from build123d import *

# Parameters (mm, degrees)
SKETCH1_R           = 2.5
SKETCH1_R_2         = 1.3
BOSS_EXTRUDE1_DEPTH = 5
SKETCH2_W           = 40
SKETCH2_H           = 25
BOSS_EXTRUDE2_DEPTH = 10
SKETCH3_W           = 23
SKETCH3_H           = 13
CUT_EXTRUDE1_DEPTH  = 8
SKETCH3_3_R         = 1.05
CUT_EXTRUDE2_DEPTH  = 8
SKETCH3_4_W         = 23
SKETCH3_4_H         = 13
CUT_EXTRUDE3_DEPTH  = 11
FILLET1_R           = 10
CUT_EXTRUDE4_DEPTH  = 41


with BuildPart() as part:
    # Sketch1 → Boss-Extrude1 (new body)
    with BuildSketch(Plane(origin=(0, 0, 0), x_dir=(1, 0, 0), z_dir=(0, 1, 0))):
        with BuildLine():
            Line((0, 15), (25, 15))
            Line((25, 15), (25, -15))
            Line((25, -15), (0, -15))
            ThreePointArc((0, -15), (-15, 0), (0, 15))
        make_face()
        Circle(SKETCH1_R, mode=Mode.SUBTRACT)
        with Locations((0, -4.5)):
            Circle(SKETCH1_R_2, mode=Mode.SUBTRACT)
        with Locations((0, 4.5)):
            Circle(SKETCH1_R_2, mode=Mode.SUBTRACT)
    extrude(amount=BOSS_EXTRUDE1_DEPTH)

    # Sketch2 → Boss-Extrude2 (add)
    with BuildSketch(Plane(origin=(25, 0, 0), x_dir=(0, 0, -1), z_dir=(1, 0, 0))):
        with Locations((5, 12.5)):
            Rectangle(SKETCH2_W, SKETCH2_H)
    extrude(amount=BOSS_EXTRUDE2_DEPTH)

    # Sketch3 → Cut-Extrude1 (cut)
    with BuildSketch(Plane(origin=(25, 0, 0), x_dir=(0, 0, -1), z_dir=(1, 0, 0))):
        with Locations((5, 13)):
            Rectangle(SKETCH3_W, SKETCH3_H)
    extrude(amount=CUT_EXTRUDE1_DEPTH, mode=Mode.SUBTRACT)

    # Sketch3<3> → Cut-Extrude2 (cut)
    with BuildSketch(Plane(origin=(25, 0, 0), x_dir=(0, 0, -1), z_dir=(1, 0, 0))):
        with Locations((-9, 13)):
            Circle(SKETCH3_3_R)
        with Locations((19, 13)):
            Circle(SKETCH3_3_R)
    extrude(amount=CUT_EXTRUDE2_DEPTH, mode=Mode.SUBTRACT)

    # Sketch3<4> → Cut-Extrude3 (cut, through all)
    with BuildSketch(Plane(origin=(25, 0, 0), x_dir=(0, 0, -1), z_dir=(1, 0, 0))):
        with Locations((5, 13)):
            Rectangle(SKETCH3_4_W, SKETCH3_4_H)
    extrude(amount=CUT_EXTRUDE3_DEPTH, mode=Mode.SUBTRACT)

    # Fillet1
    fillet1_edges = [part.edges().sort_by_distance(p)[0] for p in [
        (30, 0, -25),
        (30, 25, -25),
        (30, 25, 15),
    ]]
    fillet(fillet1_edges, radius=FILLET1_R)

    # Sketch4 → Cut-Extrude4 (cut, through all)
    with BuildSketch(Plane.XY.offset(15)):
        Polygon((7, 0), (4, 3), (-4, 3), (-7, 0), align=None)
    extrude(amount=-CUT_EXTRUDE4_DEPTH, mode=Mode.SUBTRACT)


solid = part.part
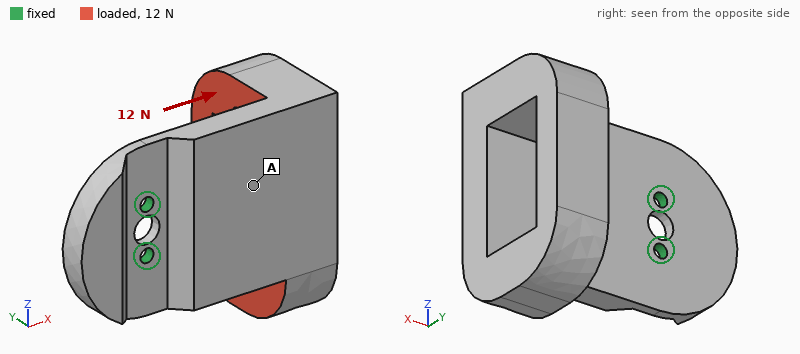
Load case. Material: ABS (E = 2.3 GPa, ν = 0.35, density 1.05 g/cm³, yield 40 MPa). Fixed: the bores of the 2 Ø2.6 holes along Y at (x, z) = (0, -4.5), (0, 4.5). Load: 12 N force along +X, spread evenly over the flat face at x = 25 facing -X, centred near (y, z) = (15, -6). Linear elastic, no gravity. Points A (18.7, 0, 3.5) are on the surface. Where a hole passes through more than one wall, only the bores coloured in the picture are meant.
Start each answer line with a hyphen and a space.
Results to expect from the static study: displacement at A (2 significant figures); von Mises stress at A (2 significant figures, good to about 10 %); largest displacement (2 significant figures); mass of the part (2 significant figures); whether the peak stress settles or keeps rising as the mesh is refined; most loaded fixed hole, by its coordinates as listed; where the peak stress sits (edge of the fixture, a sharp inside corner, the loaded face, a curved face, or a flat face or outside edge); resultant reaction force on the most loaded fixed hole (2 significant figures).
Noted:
- 0.28 mm
- 0.98 MPa
- 0.74 mm
- 11 g
- keeps rising
- (0, -4.5)
- edge of the fixture
- 13 N
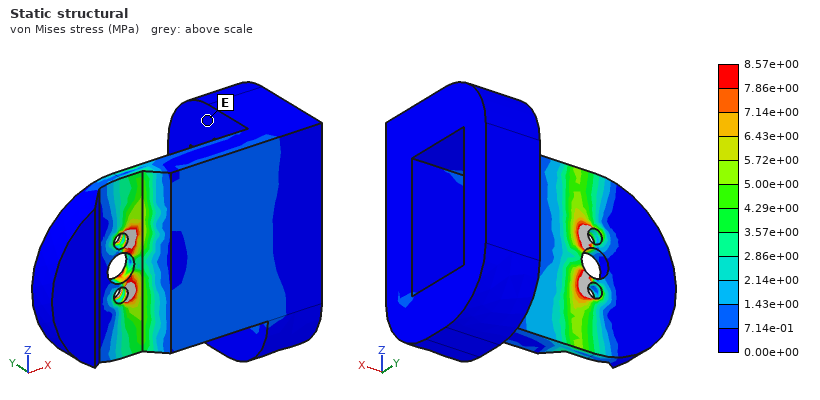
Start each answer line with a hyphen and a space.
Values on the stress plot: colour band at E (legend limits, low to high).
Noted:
- 0.00e+00 to 7.14e-01 MPa
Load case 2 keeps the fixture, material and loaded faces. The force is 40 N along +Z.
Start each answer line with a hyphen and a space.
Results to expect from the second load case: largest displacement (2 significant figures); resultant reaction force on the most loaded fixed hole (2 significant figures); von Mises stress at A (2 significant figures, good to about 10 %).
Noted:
- 0.78 mm
- 97 N
- 3.1 MPa
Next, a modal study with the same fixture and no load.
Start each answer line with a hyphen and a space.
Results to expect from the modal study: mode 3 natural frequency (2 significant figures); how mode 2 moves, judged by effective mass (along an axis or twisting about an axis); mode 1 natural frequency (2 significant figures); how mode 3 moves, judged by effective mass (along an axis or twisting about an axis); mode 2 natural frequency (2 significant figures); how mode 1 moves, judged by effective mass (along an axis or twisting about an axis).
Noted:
- 1100 Hz
- along Z
- 170 Hz
- along Z
- 480 Hz
- along Y
